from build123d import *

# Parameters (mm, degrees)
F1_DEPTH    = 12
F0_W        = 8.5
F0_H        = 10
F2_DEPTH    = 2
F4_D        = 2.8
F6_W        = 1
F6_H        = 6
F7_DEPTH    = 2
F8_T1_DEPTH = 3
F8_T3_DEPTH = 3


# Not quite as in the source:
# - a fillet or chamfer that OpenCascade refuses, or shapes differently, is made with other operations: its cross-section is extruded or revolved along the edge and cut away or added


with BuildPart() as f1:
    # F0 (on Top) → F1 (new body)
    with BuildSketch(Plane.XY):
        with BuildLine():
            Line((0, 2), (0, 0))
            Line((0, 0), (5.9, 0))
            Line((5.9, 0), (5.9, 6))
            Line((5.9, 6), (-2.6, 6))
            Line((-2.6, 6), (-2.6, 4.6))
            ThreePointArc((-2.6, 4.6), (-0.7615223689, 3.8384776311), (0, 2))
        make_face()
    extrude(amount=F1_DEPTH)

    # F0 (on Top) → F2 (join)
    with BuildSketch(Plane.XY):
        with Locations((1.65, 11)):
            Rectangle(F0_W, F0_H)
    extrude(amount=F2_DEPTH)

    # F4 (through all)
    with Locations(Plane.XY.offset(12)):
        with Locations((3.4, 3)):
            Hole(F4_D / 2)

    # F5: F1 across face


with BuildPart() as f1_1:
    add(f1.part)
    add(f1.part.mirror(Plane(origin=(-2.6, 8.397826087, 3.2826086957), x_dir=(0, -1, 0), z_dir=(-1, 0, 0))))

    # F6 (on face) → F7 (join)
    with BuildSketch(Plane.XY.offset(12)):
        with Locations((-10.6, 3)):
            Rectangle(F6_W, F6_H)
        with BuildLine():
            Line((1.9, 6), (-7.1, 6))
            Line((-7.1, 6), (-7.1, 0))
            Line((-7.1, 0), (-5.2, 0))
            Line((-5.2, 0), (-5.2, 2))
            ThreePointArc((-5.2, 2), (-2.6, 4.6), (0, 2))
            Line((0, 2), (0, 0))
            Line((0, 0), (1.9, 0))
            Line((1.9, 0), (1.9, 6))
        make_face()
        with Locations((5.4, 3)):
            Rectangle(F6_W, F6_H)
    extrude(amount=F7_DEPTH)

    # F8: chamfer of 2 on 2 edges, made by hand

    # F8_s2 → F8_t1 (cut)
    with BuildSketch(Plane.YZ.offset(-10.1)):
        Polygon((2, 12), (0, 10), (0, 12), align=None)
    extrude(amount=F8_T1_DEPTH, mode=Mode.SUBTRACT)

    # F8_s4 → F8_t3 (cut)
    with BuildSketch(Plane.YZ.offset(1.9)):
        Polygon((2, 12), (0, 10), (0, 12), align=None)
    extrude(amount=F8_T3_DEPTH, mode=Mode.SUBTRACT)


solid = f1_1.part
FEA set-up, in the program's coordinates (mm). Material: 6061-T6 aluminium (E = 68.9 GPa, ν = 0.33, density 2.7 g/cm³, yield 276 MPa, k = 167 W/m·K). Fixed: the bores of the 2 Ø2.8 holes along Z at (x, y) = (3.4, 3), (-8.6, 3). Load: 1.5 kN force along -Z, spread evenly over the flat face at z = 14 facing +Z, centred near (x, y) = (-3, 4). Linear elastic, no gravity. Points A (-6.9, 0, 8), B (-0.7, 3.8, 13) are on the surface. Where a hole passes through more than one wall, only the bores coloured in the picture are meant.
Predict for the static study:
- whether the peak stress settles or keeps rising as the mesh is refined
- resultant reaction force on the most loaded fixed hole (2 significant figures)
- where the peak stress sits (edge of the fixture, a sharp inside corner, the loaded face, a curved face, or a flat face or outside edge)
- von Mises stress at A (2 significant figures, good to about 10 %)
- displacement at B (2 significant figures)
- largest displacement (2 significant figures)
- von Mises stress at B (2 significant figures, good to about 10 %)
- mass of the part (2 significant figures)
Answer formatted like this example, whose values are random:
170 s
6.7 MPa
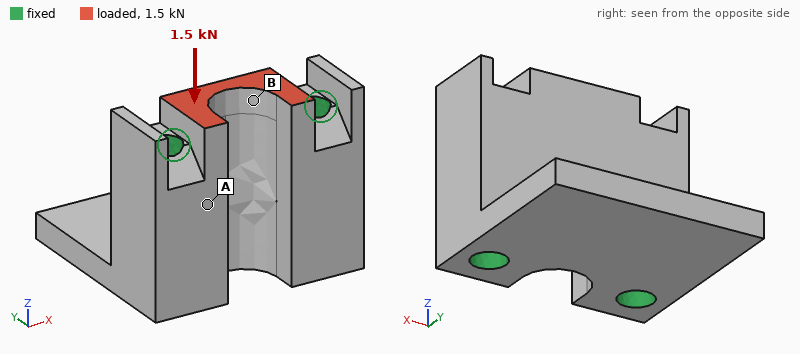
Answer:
keeps rising
760 N
edge of the fixture
14 MPa
4.0 µm
6.1 µm
41 MPa
3.4 g
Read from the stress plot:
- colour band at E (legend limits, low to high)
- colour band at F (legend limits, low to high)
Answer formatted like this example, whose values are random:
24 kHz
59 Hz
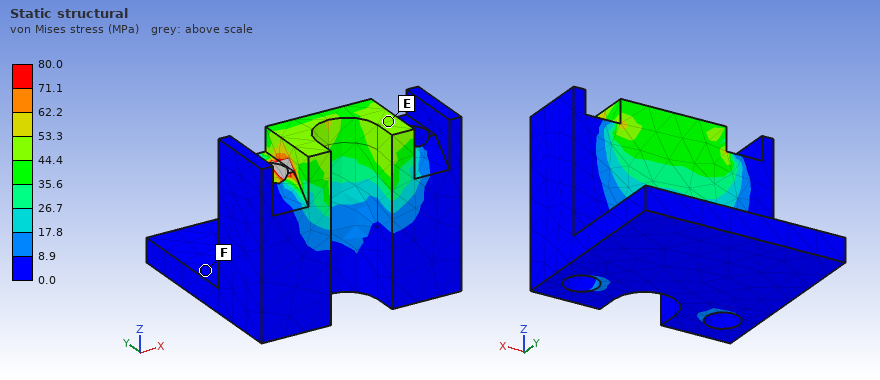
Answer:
44.4 to 53.3 MPa
0.0 to 8.9 MPa
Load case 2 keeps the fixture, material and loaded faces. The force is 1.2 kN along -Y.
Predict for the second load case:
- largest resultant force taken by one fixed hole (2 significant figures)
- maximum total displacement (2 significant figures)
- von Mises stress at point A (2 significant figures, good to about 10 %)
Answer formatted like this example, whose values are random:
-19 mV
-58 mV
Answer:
610 N
22 µm
47 MPa
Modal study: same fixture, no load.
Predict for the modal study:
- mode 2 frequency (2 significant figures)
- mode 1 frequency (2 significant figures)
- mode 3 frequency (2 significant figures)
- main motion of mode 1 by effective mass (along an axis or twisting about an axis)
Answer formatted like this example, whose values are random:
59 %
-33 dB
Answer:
23 kHz
13 kHz
49 kHz
along Z
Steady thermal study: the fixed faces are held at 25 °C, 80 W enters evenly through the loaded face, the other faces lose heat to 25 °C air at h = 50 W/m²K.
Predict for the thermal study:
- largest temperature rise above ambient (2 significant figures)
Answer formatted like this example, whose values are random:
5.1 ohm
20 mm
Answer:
65 K
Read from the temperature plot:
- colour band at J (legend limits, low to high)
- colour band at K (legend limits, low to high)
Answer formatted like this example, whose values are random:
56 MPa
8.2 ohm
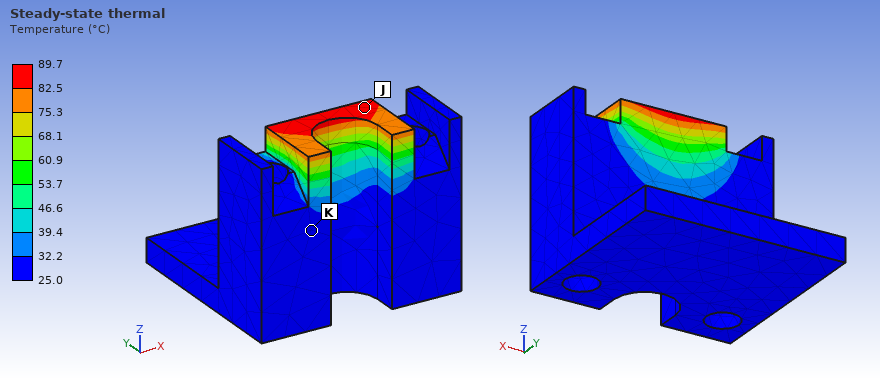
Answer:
82.5 to 89.7 °C
25.0 to 32.2 °C
